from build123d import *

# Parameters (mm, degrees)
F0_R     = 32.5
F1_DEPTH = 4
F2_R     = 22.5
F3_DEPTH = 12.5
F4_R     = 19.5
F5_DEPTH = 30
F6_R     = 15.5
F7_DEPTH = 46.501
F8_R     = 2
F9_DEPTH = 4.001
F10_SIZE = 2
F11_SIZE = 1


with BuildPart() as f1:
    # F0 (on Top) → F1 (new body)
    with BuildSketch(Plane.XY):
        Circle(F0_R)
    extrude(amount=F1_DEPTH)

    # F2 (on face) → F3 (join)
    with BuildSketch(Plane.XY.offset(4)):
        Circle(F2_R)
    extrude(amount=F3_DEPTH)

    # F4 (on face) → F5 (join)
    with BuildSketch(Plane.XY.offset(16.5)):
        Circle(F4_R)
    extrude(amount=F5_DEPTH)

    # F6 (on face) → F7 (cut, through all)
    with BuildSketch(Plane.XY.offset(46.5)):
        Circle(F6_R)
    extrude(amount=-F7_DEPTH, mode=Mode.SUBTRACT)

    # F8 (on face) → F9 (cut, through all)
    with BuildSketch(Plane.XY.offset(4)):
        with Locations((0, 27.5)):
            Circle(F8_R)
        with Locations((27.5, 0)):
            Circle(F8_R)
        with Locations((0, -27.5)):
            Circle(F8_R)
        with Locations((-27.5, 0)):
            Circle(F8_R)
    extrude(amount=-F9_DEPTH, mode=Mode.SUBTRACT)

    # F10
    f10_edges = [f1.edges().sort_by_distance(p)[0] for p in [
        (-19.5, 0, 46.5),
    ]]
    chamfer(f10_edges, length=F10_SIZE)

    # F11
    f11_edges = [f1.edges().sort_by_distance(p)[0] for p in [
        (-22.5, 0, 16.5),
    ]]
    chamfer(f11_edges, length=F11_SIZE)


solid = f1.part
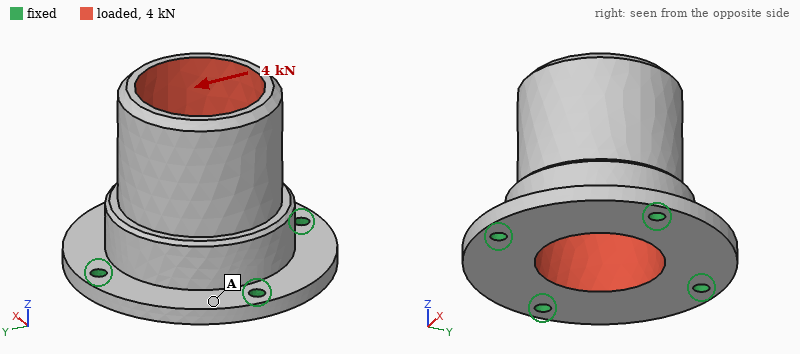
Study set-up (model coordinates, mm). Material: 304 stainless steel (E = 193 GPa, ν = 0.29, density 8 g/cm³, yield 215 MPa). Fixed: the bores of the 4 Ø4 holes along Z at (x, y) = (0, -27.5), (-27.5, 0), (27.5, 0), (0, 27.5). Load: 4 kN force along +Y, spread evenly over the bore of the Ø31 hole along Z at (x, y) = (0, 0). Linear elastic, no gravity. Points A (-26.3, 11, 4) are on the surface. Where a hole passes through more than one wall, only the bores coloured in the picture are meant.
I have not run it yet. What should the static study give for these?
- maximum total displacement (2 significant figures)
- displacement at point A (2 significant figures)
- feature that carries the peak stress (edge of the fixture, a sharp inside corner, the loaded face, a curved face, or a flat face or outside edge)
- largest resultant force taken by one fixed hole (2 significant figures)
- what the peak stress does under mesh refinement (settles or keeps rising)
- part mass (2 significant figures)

17 µm
2.7 µm
edge of the fixture
2.1 kN
keeps rising
270 g
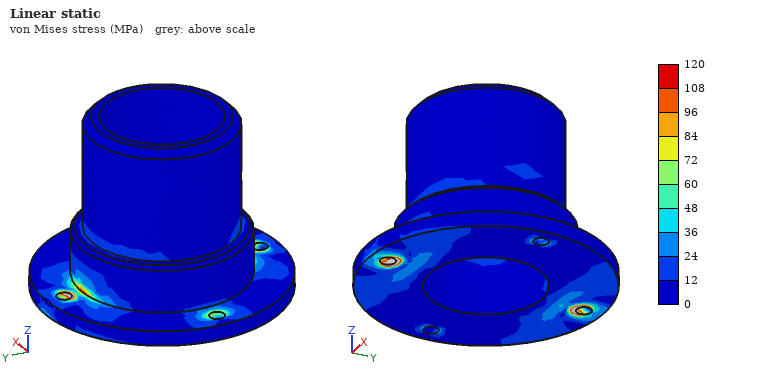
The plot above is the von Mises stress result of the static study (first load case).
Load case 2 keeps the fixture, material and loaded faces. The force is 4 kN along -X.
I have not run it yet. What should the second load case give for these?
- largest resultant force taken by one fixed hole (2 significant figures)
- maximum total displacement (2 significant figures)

2.1 kN
17 µm
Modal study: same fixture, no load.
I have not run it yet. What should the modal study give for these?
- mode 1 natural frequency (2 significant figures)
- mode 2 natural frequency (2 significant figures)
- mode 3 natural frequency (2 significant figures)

6700 Hz
6700 Hz
9300 Hz
